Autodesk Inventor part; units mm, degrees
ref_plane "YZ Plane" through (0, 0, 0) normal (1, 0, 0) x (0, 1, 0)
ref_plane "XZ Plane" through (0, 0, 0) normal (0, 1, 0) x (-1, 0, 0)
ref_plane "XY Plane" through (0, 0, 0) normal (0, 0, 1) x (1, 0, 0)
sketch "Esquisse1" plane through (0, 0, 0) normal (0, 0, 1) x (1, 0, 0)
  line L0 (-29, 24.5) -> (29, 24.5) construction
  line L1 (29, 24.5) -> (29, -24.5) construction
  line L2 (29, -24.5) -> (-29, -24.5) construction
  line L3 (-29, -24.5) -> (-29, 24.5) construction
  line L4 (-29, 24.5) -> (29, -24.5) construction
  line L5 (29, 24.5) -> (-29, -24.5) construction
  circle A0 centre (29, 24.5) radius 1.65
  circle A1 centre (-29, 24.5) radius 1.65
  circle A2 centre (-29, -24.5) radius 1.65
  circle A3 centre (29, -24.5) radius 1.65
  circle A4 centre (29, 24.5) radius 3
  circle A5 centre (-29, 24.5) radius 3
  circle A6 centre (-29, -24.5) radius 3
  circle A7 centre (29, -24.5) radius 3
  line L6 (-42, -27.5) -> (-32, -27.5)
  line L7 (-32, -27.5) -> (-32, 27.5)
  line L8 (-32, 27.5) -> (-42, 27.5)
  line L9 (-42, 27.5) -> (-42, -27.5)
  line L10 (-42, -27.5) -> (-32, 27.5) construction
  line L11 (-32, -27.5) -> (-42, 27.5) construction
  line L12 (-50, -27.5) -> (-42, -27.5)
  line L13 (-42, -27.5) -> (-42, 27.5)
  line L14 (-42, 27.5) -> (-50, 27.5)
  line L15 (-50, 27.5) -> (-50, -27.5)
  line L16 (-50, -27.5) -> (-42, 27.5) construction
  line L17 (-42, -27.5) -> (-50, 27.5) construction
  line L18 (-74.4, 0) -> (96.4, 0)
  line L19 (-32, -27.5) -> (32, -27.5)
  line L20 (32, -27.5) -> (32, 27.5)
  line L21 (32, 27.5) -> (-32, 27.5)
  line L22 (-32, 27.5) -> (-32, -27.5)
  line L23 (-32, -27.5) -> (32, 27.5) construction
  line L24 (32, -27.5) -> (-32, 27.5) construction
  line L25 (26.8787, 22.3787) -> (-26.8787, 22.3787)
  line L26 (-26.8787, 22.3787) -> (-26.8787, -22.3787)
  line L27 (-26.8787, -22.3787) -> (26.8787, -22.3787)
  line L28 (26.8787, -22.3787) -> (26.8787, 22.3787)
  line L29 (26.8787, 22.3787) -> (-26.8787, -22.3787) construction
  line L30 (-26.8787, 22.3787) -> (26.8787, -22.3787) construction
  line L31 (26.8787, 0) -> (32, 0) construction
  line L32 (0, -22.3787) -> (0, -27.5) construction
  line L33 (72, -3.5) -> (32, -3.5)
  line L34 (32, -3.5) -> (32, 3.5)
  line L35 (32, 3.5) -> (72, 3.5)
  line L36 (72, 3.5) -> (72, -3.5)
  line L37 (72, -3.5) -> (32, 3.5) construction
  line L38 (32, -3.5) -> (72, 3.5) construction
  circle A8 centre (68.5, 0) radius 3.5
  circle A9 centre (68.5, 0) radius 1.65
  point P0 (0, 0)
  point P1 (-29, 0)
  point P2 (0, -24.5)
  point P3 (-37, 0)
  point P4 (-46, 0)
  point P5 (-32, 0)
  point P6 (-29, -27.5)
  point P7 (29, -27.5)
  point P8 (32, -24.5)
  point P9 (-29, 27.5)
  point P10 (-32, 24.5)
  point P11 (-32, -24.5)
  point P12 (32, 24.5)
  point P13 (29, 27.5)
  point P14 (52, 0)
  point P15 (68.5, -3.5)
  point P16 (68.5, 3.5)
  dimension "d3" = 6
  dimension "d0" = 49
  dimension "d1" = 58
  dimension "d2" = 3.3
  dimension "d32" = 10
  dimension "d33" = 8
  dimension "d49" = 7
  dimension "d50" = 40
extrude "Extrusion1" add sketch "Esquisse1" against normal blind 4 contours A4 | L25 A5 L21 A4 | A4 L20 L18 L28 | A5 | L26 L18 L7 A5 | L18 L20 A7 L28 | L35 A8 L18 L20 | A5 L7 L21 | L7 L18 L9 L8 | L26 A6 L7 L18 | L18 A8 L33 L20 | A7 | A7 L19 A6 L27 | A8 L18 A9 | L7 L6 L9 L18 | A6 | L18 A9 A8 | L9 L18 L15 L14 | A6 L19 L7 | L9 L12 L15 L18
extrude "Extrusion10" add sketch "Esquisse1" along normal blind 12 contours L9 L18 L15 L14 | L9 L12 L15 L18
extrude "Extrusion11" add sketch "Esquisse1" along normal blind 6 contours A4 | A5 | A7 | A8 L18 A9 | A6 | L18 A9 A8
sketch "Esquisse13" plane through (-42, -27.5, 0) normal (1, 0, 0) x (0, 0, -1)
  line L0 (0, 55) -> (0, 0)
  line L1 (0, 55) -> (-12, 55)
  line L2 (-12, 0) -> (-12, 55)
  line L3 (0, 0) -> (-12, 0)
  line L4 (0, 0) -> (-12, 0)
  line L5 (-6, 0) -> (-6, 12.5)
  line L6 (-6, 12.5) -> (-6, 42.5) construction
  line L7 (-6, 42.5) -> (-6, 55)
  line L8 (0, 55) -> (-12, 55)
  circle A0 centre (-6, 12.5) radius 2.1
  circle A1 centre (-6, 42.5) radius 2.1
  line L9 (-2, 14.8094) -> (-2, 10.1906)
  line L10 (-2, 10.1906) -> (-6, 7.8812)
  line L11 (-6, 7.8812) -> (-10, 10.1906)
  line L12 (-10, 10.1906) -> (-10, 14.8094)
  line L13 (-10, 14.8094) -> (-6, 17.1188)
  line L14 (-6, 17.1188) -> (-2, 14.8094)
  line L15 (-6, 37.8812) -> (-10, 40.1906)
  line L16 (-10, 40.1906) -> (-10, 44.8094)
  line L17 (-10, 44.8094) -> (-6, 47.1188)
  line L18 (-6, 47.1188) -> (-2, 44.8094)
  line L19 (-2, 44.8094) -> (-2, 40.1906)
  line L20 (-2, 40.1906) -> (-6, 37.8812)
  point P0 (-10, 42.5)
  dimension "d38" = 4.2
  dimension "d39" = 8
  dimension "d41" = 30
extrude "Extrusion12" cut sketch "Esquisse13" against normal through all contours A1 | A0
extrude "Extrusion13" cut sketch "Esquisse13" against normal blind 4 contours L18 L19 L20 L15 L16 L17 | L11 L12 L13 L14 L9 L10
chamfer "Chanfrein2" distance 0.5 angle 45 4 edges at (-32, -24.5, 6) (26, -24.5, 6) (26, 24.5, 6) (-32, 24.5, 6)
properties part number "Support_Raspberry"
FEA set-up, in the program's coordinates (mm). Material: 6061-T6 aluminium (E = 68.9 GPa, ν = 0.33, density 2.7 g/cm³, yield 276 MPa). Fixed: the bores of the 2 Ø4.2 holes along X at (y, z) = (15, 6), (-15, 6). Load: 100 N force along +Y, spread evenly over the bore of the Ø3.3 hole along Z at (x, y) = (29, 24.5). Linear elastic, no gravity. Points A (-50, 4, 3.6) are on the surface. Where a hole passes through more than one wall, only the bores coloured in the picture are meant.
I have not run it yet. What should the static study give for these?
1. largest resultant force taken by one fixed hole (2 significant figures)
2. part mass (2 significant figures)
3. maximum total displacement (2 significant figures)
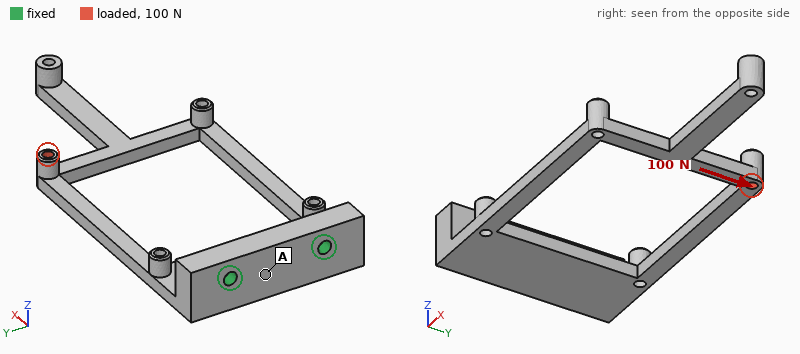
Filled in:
240 N
40 g
0.51 mm
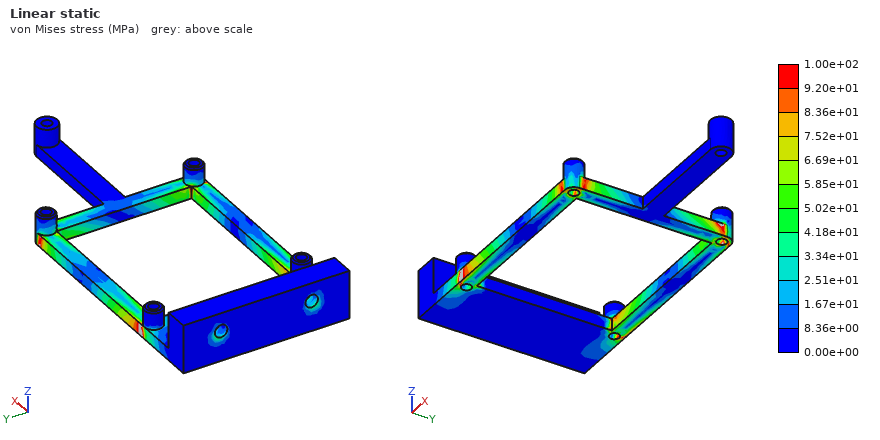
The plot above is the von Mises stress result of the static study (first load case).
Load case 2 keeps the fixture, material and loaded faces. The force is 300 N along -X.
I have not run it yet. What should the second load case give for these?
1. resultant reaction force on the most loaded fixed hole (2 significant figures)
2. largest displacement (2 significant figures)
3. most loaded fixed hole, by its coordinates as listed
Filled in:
380 N
1.1 mm
(15, 6)
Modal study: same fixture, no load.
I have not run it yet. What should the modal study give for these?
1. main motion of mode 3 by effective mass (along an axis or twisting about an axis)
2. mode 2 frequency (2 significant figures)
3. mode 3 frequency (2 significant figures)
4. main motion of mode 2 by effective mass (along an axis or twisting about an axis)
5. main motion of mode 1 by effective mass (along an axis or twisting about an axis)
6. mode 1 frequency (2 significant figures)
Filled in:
twisting about X
810 Hz
1100 Hz
along Y
along Z
270 Hz
